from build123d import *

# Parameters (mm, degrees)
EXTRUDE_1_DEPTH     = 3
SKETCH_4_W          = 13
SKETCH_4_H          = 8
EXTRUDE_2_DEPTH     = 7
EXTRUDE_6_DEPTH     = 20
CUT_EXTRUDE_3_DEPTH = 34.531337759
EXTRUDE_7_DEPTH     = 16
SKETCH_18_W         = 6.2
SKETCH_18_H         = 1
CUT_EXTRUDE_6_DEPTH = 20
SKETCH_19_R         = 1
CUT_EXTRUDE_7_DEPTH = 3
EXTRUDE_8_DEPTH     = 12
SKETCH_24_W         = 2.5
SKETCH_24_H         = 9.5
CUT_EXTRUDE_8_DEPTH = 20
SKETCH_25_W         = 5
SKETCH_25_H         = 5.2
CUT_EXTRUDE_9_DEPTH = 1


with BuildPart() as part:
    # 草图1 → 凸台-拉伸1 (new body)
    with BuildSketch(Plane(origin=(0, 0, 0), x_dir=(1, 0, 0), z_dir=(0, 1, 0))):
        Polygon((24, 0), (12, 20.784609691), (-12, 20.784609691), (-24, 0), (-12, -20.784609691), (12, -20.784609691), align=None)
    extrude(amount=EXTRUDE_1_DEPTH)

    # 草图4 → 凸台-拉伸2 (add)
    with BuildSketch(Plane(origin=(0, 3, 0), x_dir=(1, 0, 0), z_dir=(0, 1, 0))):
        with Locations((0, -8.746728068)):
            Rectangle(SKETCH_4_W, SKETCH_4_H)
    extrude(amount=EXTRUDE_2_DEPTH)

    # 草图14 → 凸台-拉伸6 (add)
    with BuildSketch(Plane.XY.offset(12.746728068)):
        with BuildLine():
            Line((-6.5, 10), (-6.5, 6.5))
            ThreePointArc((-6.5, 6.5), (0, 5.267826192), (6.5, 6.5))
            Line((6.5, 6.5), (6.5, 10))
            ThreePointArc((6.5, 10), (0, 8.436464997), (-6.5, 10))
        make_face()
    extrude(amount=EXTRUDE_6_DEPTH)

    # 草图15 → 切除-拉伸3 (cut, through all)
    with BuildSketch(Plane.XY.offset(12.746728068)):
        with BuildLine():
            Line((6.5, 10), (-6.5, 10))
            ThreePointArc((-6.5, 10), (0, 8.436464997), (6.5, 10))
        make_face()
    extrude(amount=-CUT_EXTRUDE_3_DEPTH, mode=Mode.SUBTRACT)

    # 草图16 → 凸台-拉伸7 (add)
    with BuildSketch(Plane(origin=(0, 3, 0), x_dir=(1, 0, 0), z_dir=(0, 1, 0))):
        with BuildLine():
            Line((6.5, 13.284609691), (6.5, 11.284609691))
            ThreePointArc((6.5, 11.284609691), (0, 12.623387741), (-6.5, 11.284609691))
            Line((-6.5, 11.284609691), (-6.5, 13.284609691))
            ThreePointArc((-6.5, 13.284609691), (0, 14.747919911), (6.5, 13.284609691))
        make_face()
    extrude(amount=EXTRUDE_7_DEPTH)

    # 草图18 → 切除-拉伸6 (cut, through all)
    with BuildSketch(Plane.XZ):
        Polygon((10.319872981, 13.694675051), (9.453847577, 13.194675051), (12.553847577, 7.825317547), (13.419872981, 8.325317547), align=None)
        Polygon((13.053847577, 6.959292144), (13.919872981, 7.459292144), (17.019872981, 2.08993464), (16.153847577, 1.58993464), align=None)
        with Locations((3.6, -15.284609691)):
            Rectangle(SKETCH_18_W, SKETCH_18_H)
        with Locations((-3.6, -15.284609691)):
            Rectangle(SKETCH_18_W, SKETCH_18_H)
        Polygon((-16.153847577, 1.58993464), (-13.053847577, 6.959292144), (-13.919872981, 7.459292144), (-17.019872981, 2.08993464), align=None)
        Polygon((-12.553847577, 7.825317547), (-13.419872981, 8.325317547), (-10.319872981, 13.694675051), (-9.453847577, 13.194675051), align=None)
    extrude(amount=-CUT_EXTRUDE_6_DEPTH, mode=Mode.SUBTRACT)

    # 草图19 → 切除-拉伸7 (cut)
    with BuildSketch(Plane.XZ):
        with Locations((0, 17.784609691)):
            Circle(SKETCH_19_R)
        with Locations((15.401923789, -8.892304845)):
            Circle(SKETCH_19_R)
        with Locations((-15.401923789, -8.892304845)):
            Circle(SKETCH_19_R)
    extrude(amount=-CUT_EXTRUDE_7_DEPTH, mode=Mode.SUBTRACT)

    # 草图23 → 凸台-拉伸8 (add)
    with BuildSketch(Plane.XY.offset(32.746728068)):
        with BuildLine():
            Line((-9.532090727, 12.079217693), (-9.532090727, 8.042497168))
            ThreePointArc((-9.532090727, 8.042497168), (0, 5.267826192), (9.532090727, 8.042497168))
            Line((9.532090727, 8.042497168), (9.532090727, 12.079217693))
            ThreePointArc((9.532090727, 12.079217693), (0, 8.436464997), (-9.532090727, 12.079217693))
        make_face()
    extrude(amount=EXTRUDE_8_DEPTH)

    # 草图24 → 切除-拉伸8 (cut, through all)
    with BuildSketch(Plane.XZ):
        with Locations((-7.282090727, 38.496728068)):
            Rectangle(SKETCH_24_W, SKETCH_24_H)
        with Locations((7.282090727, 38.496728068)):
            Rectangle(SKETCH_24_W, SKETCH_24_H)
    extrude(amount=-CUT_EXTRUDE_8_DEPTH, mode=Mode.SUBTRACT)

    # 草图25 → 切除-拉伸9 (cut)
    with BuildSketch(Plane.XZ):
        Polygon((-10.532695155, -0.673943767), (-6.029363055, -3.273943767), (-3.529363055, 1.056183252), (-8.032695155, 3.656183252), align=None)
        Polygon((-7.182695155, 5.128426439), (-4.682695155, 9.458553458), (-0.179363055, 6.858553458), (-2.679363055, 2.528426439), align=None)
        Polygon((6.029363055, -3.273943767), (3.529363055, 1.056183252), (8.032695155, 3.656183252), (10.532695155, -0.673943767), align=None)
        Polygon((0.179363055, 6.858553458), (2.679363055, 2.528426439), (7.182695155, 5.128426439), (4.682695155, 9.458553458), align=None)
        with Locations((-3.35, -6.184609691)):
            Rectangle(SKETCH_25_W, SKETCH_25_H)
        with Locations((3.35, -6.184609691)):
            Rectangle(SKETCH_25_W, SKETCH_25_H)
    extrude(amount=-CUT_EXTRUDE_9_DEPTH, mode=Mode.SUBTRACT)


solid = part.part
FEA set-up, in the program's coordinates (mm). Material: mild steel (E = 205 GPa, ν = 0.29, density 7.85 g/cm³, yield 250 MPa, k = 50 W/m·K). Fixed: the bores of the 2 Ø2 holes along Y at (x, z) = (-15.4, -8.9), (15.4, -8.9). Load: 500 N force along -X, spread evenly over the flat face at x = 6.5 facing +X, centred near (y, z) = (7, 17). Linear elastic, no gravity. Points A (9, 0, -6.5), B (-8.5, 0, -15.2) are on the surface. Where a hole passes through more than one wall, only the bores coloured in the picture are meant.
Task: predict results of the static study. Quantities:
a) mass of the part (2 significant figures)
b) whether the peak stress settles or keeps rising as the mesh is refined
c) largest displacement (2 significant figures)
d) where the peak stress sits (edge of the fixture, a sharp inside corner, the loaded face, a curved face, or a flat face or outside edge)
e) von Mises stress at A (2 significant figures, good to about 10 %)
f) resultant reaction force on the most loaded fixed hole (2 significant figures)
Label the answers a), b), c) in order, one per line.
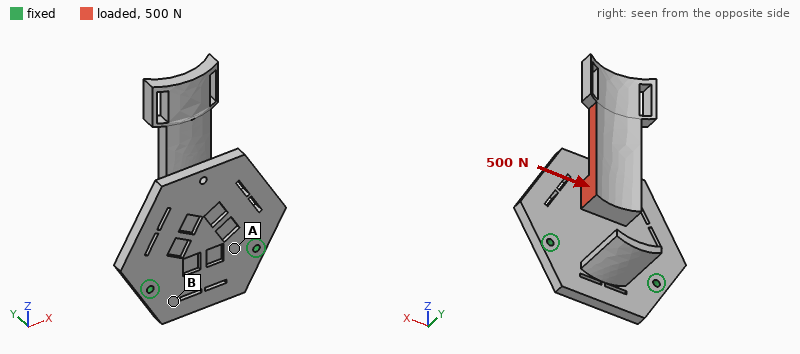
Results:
a) 53 g
b) keeps rising
c) 32 µm
d) edge of the fixture
e) 16 MPa
f) 490 N
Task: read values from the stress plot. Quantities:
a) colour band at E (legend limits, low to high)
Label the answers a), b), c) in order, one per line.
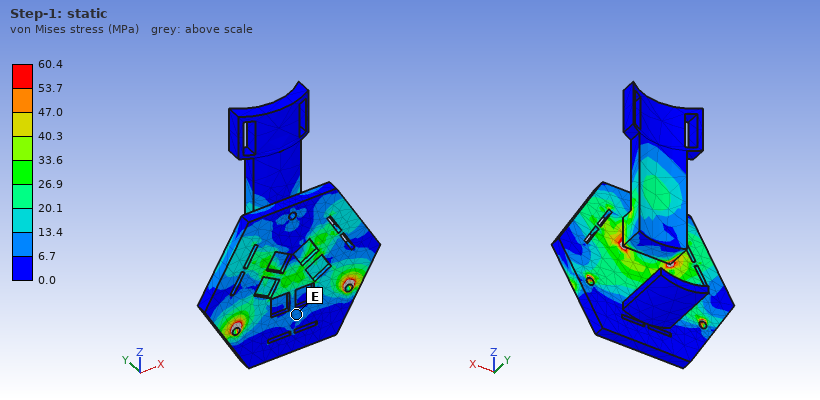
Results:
a) 6.7 to 13.4 MPa
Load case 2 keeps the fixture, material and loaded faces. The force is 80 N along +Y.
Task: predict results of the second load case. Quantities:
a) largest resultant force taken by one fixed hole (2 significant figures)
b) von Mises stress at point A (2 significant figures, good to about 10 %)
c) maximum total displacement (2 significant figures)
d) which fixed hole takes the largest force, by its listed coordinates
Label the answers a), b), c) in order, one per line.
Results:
a) 59 N
b) 26 MPa
c) 0.10 mm
d) (15.4, -8.9)
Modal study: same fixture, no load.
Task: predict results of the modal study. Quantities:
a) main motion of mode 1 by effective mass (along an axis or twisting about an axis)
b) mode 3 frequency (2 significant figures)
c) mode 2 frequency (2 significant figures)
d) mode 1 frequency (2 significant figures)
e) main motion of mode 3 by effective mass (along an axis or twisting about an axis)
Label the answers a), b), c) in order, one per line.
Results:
a) along Y
b) 4900 Hz
c) 3900 Hz
d) 1000 Hz
e) along X
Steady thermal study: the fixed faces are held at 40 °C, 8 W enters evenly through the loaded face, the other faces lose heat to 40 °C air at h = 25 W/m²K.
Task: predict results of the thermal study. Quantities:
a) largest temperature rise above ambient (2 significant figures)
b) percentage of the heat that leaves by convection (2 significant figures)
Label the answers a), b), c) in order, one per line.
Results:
a) 50 K
b) 35 %
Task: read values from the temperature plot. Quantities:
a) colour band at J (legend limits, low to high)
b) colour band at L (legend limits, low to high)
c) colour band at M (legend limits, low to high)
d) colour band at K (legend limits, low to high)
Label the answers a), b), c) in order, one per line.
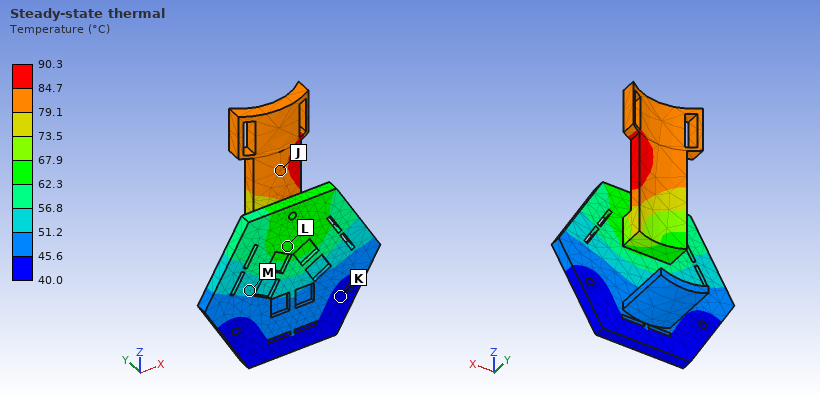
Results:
a) 79.1 to 84.7 °C
b) 62.3 to 67.9 °C
c) 51.2 to 56.8 °C
d) 40.0 to 45.6 °C
